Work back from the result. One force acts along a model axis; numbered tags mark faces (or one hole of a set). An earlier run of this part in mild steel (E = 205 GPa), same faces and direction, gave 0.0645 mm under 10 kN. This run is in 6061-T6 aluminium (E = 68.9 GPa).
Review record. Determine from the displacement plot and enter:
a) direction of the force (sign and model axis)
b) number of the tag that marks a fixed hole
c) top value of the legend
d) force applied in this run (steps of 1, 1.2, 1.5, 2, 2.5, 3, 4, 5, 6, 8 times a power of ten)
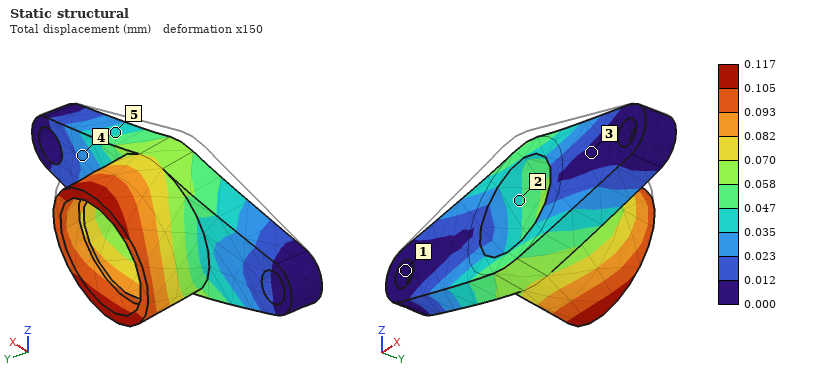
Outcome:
-Z
1
0.117 mm
6 kN
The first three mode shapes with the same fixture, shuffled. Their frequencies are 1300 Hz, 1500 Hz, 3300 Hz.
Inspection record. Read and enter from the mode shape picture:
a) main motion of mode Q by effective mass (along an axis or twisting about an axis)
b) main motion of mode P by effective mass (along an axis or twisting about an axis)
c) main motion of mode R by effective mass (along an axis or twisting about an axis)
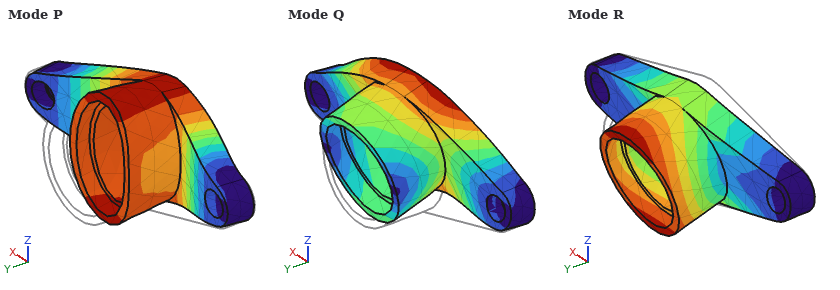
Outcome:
along Z
along Y
along Z
